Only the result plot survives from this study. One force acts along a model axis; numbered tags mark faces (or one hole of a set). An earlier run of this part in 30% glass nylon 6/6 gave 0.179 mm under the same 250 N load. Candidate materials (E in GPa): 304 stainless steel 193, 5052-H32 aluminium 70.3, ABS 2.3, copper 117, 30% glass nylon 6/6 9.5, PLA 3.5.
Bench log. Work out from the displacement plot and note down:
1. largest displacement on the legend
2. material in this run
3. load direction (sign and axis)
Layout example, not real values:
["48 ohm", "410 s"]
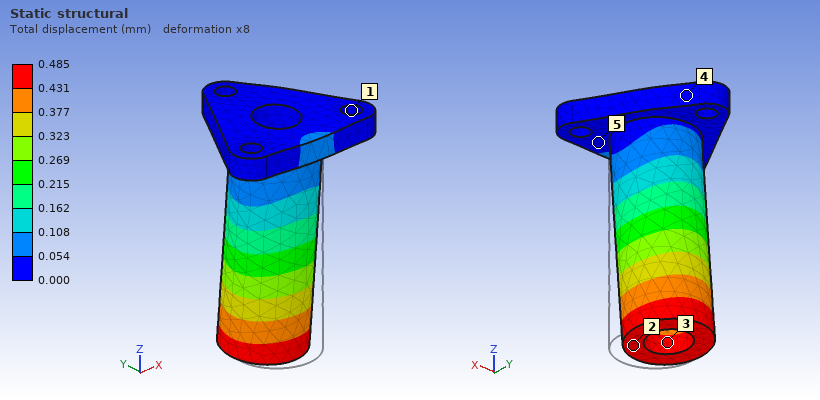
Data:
["0.485 mm", "PLA", "+Y"]
